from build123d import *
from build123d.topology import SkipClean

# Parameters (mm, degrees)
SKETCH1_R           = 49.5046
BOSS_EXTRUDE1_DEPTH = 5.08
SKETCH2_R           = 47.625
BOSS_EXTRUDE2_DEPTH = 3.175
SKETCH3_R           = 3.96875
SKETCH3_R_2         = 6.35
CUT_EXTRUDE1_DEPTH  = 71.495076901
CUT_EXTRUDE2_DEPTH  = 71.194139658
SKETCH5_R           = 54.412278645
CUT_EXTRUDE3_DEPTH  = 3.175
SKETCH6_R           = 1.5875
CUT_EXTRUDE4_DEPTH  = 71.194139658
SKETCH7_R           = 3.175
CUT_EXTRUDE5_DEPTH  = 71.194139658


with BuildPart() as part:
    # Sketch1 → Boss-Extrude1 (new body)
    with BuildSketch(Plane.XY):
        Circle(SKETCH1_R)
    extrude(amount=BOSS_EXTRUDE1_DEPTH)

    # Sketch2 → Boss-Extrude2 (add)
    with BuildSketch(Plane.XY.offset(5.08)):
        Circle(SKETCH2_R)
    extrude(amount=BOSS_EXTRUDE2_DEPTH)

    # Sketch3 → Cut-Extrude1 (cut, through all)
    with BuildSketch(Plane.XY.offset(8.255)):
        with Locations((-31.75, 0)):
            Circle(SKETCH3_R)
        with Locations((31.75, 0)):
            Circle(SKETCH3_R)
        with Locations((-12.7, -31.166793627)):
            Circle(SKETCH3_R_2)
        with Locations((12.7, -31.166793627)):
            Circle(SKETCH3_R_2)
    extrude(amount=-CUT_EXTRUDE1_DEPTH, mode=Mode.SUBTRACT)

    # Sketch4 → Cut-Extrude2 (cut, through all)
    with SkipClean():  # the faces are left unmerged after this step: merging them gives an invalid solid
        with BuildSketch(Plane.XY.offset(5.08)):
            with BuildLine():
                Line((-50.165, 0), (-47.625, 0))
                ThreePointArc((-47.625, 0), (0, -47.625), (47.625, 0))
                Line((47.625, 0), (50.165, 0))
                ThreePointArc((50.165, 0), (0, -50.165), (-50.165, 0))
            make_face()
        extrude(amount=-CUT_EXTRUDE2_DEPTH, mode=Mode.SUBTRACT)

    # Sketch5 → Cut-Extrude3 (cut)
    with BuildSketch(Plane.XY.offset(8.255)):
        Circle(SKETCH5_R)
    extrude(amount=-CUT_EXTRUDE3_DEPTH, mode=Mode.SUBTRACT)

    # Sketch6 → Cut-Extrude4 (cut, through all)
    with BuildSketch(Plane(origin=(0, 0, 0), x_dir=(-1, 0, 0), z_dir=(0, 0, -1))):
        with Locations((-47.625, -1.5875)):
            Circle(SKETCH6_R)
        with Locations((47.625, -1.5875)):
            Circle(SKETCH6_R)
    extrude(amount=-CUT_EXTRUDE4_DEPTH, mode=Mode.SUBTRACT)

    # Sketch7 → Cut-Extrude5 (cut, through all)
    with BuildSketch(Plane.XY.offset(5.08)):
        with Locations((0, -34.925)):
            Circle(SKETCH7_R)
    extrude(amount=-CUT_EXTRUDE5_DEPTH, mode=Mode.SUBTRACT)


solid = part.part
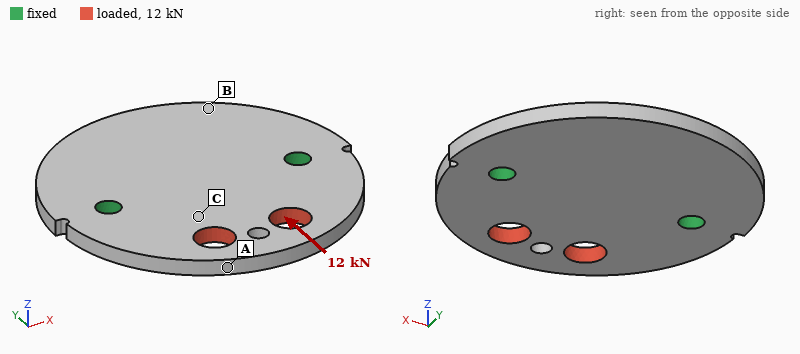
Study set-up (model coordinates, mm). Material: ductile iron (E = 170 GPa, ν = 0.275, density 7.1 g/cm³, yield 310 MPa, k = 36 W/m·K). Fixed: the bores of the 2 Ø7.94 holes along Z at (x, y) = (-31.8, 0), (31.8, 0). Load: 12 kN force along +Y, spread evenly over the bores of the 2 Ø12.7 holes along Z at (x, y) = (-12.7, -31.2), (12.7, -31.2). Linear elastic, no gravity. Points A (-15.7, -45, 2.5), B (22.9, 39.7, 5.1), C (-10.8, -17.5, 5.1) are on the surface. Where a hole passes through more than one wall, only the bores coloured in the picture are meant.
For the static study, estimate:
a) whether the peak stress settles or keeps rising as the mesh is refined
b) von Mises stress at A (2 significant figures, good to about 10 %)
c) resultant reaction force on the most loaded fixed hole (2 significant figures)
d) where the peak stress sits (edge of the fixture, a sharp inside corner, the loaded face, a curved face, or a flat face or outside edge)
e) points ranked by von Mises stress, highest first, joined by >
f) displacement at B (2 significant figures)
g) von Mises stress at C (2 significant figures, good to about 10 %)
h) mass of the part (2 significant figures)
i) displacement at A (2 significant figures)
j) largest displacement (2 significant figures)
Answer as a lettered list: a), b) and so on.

a) keeps rising
b) 53 MPa
c) 6.1 kN
d) edge of the fixture
e) A > C > B
f) 3.1 µm
g) 38 MPa
h) 250 g
i) 13 µm
j) 15 µm
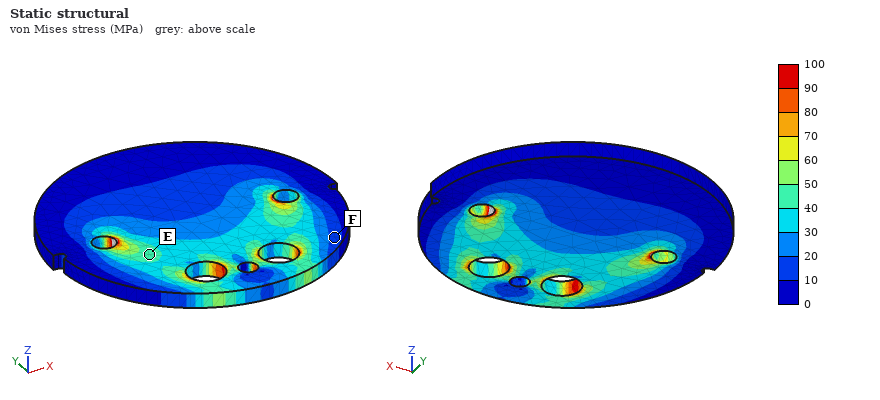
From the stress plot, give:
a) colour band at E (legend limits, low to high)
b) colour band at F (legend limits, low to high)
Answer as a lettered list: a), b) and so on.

a) 40 to 50 MPa
b) 10 to 20 MPa
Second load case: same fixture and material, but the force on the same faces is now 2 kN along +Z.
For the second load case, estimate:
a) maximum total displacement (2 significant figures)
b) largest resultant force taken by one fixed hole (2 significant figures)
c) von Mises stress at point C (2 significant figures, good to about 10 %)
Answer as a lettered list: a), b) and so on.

a) 0.31 mm
b) 1.0 kN
c) 84 MPa
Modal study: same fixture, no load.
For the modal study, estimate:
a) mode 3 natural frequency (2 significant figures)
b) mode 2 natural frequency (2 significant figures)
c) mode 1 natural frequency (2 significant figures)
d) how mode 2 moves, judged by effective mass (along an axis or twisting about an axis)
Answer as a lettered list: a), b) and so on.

a) 4500 Hz
b) 2400 Hz
c) 1900 Hz
d) along Z
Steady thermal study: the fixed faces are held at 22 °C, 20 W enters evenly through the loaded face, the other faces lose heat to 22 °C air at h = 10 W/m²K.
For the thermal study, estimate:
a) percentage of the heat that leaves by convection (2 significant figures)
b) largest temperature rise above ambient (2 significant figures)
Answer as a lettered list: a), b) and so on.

a) 14 %
b) 64 K
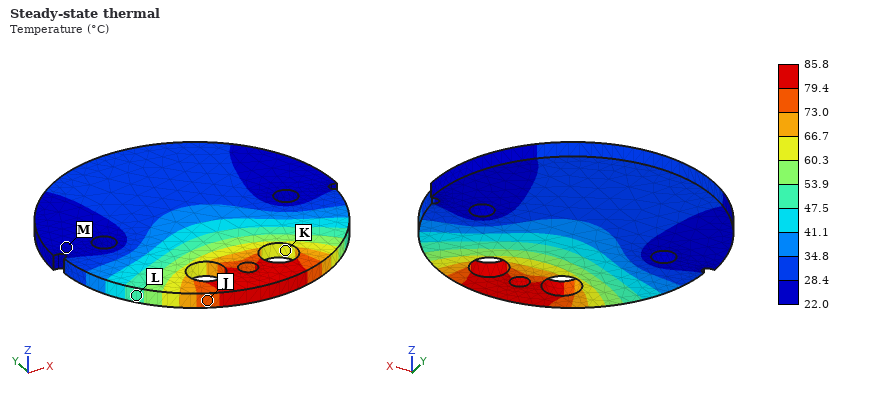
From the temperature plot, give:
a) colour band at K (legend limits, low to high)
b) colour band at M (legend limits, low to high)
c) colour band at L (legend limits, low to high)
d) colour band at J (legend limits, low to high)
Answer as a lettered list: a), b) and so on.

a) 60.3 to 66.7 °C
b) 22.0 to 28.4 °C
c) 47.5 to 53.9 °C
d) 73.0 to 79.4 °C
